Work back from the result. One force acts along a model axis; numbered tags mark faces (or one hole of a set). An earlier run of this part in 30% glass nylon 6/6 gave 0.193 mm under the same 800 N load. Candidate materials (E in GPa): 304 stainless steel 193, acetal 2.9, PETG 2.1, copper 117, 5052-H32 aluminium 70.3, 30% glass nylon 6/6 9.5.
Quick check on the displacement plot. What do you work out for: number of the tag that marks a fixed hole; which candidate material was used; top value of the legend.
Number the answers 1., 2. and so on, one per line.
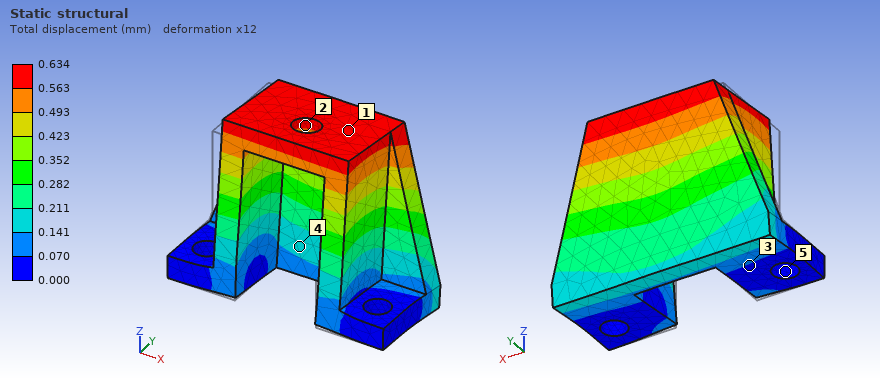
1. 5
2. acetal
3. 0.634 mm
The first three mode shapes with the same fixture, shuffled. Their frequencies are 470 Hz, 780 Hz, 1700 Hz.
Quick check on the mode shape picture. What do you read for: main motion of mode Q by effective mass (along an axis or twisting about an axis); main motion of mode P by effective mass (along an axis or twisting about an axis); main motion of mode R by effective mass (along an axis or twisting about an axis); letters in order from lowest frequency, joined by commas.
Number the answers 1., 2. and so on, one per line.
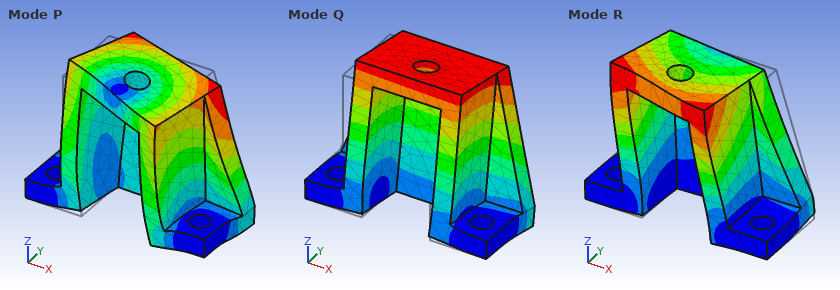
1. along Y
2. along X
3. along X
4. Q, R, P
